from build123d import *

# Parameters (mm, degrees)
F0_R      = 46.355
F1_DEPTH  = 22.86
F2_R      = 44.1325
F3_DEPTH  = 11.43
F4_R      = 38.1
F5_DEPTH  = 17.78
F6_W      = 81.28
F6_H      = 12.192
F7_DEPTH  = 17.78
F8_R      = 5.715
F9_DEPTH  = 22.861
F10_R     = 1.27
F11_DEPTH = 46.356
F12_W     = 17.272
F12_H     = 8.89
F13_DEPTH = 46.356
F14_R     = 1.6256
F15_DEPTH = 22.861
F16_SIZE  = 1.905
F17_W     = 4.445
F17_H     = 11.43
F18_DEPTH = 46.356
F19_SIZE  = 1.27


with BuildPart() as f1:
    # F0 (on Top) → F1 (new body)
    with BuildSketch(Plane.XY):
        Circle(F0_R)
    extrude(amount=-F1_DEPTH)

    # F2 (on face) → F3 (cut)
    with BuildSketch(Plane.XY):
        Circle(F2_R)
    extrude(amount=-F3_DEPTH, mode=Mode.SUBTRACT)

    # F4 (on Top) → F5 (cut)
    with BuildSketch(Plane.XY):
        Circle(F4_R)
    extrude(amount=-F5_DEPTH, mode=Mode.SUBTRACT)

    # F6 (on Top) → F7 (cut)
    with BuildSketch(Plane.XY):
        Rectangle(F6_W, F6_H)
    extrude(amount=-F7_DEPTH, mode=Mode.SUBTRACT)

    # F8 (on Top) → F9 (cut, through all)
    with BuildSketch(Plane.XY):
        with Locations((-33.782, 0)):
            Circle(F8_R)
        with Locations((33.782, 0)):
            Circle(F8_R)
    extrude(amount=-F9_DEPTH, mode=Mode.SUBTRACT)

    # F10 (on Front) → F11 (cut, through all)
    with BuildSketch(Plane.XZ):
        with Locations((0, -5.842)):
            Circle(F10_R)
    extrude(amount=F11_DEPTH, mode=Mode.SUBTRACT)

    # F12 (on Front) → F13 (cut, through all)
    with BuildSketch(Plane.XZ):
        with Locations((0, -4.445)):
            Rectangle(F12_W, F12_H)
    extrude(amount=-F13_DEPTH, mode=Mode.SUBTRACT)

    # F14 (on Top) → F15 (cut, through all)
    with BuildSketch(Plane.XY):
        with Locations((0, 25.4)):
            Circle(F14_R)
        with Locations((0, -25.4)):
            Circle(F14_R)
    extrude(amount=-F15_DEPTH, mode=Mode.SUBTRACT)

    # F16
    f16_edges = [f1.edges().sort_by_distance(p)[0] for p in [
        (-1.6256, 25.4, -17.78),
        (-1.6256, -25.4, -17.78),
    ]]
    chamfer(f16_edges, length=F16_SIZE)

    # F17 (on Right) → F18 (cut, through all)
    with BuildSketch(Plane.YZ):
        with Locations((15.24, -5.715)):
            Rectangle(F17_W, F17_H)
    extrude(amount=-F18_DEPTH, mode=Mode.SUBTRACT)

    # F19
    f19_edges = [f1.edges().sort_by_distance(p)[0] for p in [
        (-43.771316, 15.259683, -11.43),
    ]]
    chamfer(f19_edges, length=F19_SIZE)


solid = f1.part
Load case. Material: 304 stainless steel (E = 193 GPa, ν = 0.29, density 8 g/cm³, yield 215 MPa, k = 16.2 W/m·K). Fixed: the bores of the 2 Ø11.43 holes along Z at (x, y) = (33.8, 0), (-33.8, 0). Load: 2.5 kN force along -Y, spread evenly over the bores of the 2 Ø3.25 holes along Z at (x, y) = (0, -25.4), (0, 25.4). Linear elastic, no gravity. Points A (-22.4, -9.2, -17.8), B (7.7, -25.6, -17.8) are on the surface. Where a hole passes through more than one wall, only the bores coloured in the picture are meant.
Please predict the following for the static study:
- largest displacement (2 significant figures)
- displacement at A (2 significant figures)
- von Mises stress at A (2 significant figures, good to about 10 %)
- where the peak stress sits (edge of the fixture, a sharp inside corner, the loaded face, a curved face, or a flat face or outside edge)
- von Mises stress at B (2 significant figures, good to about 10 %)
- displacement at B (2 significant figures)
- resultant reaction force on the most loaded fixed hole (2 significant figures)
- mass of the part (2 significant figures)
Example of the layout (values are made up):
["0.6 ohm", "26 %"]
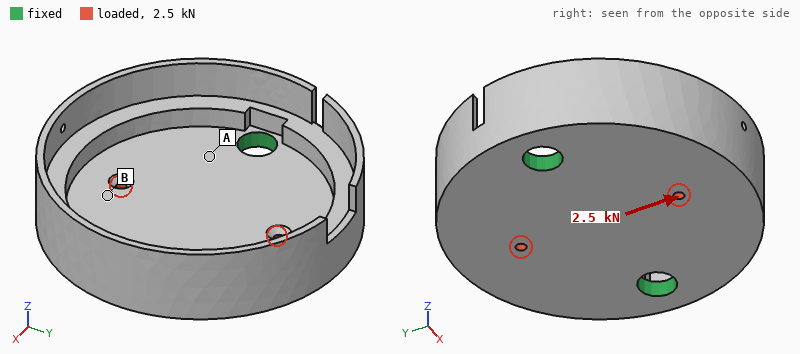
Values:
["3.2 µm", "0.57 µm", "8.0 MPa", "the loaded face", "3.9 MPa", "1.2 µm", "1.3 kN", "430 g"]
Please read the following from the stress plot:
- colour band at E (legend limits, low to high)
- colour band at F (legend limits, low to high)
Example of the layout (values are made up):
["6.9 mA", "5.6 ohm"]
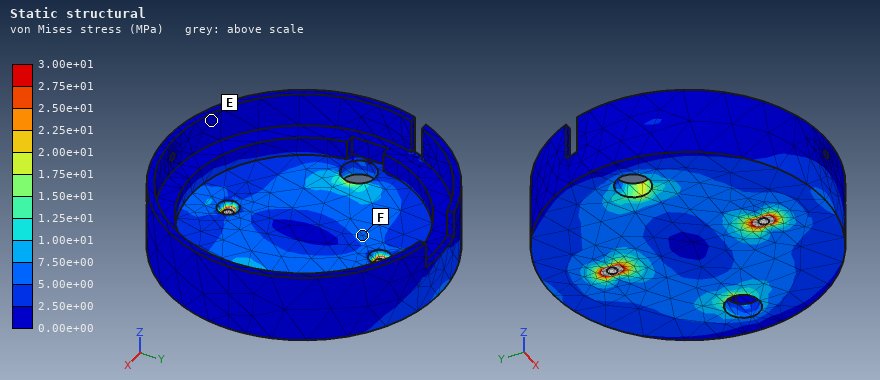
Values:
["0.00e+00 to 2.50e+00 MPa", "5.00e+00 to 7.50e+00 MPa"]
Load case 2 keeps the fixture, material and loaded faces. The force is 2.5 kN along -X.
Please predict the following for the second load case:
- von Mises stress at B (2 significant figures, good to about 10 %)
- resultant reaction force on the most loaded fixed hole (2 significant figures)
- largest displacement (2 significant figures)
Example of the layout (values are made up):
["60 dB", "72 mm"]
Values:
["7.7 MPa", "1.3 kN", "2.2 µm"]
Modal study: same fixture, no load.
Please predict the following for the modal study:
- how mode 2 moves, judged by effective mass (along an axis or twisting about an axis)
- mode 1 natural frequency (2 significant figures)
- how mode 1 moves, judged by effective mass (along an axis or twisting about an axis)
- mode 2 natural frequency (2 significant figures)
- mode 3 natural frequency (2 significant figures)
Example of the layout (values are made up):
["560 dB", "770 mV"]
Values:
["along Z", "2500 Hz", "twisting about X", "3100 Hz", "5100 Hz"]
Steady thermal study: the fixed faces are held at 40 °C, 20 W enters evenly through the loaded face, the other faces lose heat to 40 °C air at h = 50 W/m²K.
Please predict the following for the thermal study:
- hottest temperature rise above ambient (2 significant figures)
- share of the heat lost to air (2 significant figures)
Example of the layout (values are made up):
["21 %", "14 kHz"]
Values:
["70 K", "70 %"]
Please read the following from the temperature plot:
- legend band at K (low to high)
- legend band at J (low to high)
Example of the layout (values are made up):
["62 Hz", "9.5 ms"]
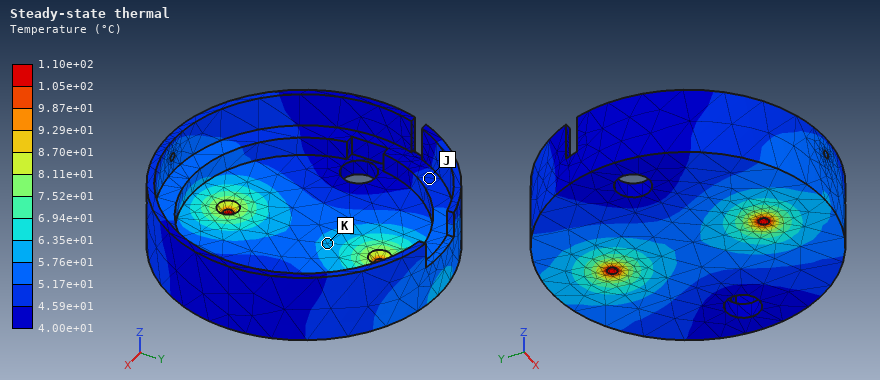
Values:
["5.76e+01 to 6.35e+01 °C", "4.59e+01 to 5.17e+01 °C"]
